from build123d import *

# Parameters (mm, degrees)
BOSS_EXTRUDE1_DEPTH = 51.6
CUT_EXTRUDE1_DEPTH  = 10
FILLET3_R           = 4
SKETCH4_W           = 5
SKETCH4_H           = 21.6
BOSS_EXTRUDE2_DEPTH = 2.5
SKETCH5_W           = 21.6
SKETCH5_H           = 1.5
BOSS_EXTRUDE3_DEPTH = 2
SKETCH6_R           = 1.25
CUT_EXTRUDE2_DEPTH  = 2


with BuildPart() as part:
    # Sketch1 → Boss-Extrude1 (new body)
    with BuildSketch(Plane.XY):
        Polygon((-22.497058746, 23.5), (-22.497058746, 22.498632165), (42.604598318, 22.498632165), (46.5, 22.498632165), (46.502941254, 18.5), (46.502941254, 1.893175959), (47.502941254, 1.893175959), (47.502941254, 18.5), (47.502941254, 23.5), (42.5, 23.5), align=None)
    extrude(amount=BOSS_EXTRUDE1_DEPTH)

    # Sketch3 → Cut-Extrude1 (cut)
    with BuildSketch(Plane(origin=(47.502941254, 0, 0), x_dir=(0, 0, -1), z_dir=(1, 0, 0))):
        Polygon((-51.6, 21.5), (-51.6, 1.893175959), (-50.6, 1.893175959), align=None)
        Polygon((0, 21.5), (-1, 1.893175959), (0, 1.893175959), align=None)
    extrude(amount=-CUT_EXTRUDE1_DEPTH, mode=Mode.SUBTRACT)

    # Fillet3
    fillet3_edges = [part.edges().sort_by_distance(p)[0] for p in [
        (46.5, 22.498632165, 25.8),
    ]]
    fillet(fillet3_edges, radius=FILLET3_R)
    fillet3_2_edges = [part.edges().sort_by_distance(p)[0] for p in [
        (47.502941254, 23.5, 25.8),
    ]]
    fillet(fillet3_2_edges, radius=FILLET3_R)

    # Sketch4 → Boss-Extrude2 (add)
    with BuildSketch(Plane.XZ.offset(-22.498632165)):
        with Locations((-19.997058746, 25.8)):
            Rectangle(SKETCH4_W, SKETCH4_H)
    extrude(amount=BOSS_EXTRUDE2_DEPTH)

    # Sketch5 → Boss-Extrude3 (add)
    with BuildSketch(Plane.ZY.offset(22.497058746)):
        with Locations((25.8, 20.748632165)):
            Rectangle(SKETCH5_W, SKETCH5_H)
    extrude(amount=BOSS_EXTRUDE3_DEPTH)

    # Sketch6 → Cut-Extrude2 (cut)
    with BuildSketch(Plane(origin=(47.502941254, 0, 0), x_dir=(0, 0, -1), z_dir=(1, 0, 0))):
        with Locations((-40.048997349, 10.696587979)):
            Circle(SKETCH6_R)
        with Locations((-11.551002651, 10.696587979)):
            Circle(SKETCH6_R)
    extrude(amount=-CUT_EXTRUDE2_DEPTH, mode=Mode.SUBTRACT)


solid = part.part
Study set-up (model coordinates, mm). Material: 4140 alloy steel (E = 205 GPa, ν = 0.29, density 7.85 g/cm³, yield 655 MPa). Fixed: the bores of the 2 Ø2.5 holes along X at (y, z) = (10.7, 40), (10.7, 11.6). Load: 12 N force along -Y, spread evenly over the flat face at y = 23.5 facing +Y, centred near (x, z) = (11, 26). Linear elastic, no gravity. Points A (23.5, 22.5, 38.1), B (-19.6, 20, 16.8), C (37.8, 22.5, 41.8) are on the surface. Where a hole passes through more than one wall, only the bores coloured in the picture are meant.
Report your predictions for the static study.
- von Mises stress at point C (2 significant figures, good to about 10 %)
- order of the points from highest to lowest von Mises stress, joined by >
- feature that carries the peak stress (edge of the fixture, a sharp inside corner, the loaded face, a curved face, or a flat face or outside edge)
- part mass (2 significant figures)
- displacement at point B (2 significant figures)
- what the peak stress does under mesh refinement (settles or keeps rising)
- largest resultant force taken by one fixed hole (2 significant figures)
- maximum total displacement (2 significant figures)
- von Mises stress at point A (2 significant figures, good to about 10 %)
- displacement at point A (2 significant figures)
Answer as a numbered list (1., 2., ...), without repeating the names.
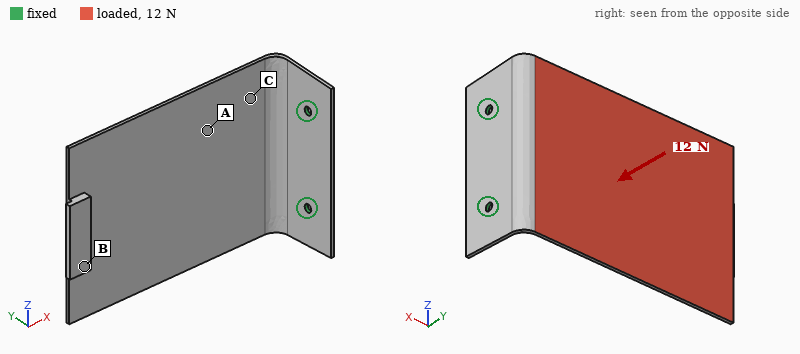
1. 34 MPa
2. C > A > B
3. edge of the fixture
4. 39 g
5. 0.82 mm
6. keeps rising
7. 6.4 N
8. 0.89 mm
9. 21 MPa
10. 0.21 mm
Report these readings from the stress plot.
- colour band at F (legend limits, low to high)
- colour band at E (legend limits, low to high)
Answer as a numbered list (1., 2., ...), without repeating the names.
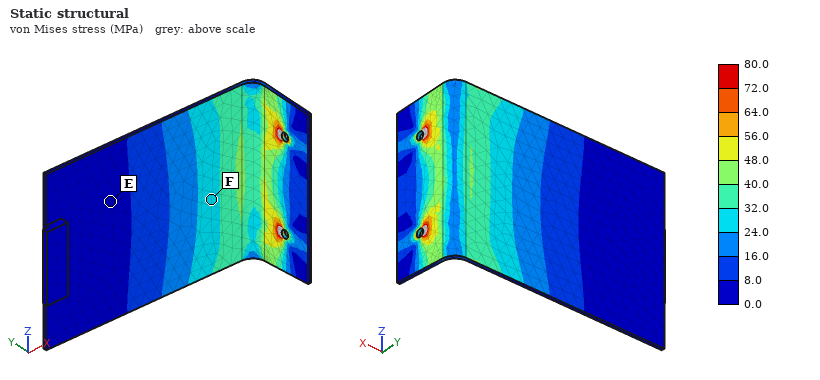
1. 24.0 to 32.0 MPa
2. 0.0 to 8.0 MPa
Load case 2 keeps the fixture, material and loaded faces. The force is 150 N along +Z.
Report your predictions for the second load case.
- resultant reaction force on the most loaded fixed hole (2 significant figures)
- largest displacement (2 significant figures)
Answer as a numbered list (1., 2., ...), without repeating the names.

1. 200 N
2. 0.74 mm
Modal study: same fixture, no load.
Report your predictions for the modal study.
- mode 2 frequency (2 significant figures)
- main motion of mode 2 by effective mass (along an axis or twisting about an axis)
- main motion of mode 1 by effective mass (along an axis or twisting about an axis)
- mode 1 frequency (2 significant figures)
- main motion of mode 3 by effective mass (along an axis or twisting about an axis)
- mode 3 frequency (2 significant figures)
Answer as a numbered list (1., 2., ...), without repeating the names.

1. 420 Hz
2. along Z
3. along Y
4. 120 Hz
5. along Z
6. 610 Hz
